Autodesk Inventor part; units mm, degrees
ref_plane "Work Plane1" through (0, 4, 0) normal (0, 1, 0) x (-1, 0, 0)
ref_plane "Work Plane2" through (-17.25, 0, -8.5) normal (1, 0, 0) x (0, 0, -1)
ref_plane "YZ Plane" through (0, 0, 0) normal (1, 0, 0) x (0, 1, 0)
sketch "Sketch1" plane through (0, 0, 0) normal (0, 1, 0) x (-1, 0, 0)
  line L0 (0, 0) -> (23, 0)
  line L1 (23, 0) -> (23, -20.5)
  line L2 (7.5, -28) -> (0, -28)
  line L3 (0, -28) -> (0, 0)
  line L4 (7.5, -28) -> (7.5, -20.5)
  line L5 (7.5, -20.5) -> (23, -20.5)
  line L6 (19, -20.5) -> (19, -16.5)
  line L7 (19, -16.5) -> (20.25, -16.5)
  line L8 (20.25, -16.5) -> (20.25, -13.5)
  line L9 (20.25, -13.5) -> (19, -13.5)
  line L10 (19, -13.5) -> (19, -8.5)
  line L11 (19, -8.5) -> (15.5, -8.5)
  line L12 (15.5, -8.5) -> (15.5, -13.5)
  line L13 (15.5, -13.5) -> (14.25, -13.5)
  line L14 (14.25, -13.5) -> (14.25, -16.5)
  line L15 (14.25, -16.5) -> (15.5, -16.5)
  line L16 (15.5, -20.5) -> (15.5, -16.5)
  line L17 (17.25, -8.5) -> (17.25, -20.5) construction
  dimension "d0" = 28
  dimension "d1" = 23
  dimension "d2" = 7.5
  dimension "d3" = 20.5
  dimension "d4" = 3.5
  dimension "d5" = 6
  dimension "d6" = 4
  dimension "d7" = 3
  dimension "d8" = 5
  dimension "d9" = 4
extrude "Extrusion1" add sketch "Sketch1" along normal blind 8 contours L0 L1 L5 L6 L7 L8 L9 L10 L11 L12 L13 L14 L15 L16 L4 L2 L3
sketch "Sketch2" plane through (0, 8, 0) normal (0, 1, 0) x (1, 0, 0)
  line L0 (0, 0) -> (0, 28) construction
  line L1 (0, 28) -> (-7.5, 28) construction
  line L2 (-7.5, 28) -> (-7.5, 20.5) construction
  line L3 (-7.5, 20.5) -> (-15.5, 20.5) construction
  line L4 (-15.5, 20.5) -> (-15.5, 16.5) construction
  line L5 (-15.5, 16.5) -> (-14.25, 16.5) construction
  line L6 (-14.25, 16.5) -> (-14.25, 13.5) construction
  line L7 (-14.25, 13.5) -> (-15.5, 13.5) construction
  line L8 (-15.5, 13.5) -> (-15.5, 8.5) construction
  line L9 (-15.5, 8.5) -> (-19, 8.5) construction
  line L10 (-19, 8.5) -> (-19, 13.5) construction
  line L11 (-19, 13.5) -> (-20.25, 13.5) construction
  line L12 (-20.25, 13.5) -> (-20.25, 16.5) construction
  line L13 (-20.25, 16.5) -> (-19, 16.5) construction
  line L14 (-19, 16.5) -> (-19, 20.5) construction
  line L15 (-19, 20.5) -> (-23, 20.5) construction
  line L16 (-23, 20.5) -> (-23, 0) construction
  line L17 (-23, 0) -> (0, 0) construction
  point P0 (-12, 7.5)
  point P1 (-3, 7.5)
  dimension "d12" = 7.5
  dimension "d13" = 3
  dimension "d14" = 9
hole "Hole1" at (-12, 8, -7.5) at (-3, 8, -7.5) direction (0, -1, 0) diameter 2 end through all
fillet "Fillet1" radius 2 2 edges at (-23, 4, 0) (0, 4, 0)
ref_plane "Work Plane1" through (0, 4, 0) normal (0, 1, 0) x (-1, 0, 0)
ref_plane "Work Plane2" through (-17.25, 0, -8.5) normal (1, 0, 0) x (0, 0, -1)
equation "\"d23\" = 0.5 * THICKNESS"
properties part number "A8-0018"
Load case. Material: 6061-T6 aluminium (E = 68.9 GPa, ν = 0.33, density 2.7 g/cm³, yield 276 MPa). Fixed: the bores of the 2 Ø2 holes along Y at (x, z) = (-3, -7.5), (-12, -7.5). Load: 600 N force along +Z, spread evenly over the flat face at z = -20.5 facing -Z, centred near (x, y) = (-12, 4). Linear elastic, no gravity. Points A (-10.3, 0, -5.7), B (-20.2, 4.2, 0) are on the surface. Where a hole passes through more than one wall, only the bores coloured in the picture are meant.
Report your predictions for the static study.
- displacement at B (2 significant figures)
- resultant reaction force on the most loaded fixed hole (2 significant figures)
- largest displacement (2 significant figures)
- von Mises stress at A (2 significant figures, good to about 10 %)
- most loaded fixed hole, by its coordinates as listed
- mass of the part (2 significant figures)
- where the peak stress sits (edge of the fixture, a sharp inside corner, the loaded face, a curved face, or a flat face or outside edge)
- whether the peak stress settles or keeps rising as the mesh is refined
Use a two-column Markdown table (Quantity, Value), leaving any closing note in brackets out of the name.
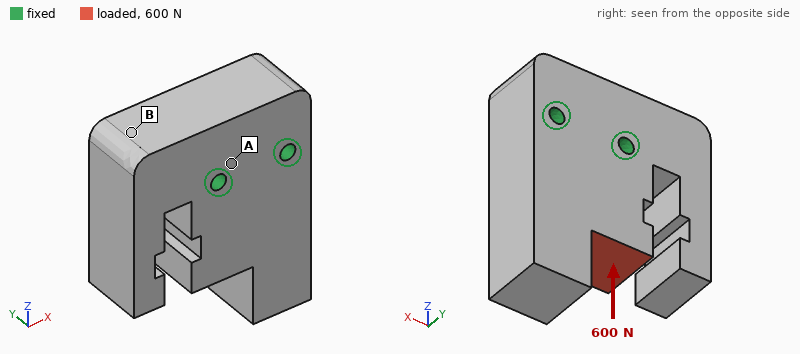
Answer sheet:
| Quantity | Value |
|---|---|
| displacement at B | 0.61 µm |
| resultant reaction force on the most loaded fixed hole | 550 N |
| largest displacement | 3.5 µm |
| von Mises stress at A | 3.9 MPa |
| most loaded fixed hole, by its coordinates as listed | (-12, -7.5) |
| mass of the part | 10 g |
| where the peak stress sits | edge of the fixture |
| whether the peak stress settles or keeps rising as the mesh is refined | keeps rising |
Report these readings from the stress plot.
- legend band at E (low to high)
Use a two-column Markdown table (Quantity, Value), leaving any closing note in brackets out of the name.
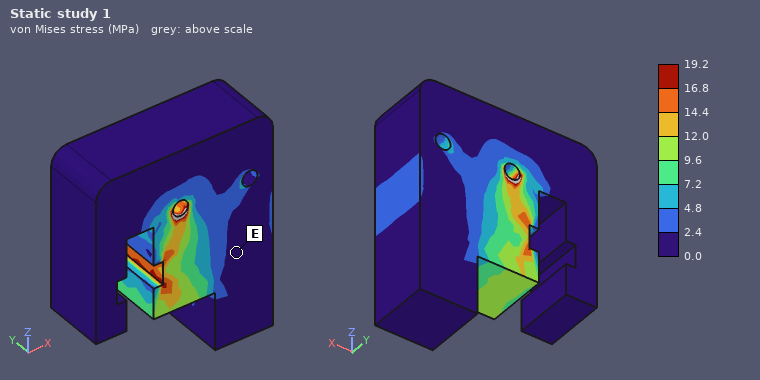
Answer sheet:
| Quantity | Value |
|---|---|
| legend band at E | 0.0 to 2.4 MPa |
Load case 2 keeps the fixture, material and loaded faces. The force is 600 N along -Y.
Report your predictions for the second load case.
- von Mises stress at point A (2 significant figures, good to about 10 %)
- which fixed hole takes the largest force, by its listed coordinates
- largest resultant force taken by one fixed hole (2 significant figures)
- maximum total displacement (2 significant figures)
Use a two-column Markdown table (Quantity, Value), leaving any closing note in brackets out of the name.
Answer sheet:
| Quantity | Value |
|---|---|
| von Mises stress at point A | 17 MPa |
| which fixed hole takes the largest force, by its listed coordinates | (-12, -7.5) |
| largest resultant force taken by one fixed hole | 470 N |
| maximum total displacement | 21 µm |
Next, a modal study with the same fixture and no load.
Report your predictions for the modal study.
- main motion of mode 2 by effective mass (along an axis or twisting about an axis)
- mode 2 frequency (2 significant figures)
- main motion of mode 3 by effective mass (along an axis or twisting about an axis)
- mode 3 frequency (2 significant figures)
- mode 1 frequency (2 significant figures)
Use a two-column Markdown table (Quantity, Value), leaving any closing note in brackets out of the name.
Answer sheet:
| Quantity | Value |
|---|---|
| main motion of mode 2 by effective mass | along Y |
| mode 2 frequency | 16 kHz |
| main motion of mode 3 by effective mass | along Y |
| mode 3 frequency | 17 kHz |
| mode 1 frequency | 13 kHz |
